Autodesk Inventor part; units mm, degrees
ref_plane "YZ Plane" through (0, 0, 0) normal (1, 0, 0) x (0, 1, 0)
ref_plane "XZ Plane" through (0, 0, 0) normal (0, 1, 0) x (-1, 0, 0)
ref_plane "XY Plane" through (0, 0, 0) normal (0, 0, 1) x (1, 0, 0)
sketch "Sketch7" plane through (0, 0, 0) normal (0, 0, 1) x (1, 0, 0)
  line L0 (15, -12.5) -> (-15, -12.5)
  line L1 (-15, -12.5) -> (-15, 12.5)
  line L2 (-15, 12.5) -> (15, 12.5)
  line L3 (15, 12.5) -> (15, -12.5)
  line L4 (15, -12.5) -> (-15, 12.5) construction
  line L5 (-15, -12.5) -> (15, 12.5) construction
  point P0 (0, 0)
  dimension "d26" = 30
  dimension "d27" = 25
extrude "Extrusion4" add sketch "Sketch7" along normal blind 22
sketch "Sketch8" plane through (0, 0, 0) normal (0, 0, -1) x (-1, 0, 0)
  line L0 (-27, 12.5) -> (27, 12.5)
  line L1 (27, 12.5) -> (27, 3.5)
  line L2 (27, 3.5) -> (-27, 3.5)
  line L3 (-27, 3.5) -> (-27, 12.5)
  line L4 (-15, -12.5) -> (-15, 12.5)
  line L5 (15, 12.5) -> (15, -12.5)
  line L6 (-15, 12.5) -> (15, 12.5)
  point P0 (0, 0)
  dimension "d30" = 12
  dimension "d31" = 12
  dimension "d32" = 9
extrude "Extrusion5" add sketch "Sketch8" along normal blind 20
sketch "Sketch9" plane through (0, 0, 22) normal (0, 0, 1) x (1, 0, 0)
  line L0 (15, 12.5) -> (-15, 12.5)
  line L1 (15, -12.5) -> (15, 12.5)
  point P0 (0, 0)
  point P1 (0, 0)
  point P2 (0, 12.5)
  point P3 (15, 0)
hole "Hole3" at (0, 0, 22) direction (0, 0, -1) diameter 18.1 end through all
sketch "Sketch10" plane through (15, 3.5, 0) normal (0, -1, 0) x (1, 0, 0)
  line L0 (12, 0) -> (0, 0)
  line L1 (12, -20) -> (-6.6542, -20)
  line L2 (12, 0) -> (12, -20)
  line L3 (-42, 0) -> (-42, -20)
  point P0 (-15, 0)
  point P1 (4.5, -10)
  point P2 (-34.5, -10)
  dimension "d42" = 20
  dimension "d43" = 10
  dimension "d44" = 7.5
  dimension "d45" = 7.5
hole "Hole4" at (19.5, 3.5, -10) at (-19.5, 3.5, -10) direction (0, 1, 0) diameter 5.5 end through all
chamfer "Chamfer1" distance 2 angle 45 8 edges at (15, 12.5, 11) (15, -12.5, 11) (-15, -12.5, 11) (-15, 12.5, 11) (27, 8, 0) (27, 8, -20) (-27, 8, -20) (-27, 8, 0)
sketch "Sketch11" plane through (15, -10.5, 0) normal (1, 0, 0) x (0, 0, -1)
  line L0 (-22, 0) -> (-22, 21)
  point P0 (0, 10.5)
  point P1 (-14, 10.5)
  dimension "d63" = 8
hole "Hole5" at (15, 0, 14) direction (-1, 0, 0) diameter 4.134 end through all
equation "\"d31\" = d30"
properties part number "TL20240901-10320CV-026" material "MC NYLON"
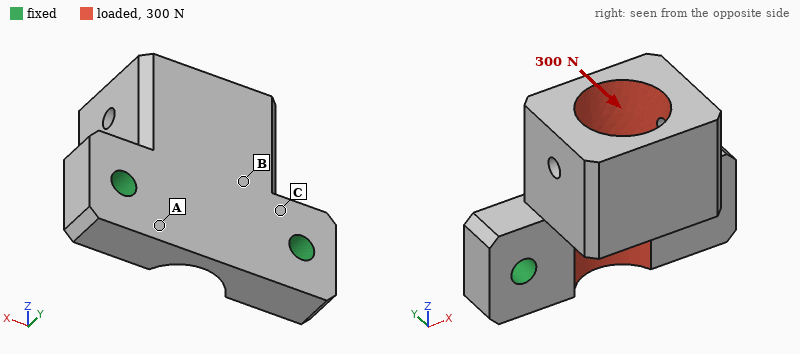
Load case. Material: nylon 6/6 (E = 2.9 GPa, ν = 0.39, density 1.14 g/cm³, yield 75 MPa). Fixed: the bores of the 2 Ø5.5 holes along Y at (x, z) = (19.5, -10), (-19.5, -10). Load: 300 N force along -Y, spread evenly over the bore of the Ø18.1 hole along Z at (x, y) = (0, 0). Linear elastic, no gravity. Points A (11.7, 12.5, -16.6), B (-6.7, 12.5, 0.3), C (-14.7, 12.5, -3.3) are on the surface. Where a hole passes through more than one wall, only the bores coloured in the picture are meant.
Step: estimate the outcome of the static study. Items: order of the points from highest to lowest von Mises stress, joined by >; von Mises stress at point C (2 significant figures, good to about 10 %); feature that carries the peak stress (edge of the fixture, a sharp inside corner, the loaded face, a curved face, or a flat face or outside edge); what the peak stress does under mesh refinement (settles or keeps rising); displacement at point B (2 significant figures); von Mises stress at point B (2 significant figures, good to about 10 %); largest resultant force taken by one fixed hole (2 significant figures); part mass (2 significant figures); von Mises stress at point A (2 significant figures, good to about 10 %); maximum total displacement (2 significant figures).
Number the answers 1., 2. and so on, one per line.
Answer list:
1. C > B > A
2. 11 MPa
3. edge of the fixture
4. keeps rising
5. 0.094 mm
6. 5.5 MPa
7. 150 N
8. 21 g
9. 2.6 MPa
10. 0.44 mm
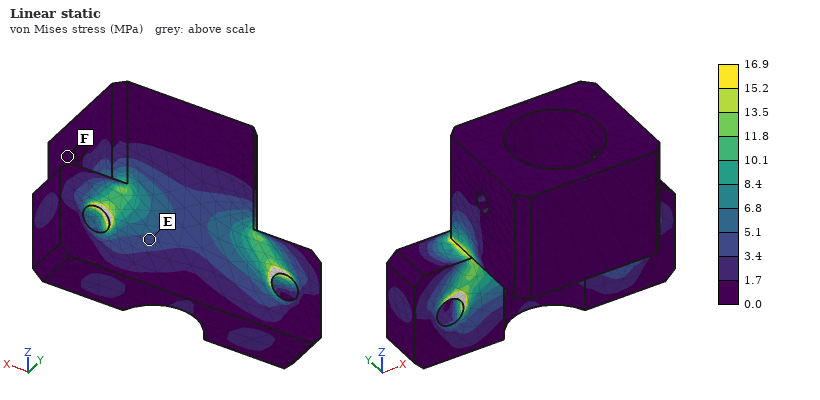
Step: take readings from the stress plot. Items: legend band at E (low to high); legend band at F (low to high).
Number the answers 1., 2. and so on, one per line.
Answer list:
1. 3.4 to 5.1 MPa
2. 0.0 to 1.7 MPa
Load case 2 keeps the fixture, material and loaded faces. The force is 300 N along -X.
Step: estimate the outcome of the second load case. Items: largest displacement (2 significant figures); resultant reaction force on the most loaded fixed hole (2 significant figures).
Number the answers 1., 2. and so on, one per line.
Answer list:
1. 84 µm
2. 190 N
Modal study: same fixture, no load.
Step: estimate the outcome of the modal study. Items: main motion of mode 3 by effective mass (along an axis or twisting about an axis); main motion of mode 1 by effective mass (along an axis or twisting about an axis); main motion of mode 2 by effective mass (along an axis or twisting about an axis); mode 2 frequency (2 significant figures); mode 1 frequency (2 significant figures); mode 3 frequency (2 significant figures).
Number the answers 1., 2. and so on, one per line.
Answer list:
1. along X
2. along Y
3. along X
4. 2500 Hz
5. 1100 Hz
6. 4100 Hz
